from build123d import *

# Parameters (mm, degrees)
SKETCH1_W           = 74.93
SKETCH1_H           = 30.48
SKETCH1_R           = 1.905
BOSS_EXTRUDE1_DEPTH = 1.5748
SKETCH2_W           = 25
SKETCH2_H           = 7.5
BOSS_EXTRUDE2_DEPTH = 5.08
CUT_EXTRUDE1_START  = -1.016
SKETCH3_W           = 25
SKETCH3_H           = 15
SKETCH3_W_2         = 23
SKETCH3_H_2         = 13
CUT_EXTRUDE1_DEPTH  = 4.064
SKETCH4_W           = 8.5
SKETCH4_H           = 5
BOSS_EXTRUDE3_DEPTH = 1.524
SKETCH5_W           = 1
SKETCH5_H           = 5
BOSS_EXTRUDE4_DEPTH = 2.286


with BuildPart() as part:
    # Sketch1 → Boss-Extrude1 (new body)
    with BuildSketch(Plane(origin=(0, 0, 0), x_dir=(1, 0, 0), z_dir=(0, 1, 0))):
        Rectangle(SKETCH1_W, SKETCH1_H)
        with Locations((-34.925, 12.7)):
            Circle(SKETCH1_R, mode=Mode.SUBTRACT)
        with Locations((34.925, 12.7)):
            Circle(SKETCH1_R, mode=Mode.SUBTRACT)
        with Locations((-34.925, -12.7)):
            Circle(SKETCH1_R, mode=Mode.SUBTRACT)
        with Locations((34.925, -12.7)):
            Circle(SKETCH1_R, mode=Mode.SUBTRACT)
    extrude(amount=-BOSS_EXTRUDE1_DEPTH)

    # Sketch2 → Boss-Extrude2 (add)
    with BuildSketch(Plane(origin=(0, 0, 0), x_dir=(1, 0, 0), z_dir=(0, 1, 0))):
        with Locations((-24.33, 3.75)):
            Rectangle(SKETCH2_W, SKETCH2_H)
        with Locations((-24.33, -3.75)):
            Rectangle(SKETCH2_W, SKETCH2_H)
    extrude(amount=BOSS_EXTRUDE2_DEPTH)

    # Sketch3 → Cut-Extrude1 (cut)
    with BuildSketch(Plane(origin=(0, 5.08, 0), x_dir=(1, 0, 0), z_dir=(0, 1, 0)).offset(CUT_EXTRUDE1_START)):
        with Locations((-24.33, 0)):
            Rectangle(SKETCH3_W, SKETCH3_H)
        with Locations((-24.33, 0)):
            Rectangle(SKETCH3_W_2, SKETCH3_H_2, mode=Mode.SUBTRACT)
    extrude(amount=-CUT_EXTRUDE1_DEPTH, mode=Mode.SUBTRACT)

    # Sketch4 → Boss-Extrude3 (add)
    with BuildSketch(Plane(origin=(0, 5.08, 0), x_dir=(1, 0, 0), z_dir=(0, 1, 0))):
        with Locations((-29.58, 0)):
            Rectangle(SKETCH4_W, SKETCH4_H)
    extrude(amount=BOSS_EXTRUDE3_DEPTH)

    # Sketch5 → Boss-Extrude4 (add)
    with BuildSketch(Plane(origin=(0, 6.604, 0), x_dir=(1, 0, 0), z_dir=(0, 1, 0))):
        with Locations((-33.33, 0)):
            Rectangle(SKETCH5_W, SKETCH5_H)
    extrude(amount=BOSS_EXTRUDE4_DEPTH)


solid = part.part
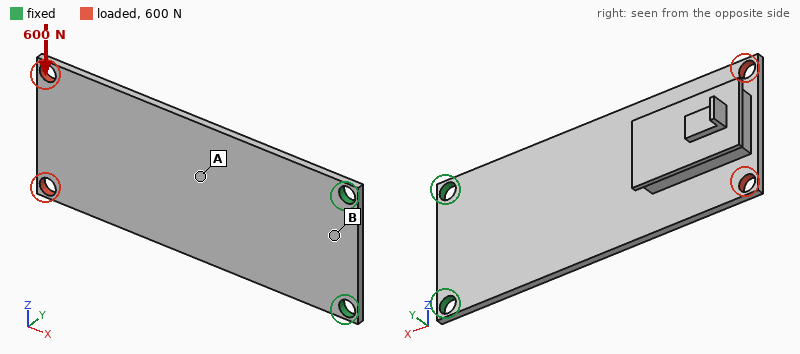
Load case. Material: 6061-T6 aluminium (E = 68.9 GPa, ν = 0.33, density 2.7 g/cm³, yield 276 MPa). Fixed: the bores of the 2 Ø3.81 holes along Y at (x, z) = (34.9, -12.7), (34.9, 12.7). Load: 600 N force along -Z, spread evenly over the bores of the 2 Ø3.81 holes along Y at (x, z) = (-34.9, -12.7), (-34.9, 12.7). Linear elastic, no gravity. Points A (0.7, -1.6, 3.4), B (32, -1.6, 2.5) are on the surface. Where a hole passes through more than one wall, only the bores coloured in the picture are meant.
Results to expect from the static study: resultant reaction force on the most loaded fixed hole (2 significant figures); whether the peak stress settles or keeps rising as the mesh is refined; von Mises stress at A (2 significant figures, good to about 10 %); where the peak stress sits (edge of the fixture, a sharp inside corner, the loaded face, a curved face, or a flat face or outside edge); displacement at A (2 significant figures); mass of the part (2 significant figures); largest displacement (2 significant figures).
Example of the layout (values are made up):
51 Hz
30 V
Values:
1.7 kN
keeps rising
37 MPa
edge of the fixture
0.096 mm
14 g
0.33 mm
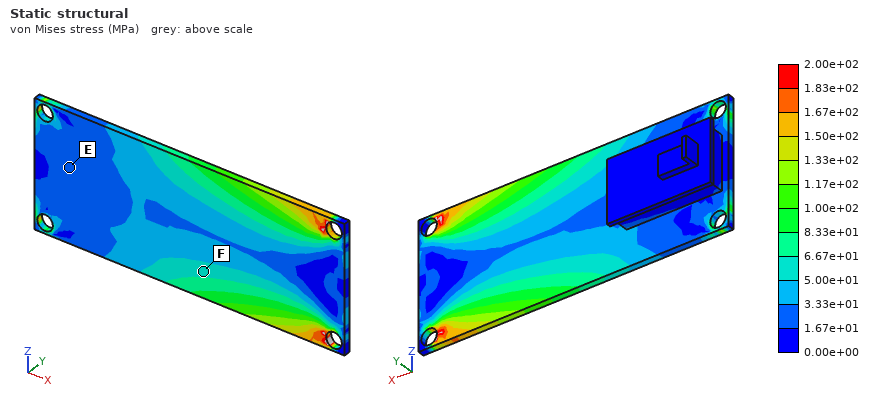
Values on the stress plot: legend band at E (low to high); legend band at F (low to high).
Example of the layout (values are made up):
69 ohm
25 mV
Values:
1.67e+01 to 3.33e+01 MPa
5.00e+01 to 6.67e+01 MPa
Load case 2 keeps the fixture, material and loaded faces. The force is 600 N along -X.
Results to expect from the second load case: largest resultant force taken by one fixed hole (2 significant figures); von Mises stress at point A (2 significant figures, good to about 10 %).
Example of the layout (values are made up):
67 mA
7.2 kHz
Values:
310 N
13 MPa
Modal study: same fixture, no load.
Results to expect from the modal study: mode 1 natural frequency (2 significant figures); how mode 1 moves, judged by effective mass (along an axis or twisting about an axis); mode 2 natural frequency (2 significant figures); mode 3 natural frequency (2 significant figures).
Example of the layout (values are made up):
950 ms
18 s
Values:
170 Hz
along Y
1200 Hz
1400 Hz
